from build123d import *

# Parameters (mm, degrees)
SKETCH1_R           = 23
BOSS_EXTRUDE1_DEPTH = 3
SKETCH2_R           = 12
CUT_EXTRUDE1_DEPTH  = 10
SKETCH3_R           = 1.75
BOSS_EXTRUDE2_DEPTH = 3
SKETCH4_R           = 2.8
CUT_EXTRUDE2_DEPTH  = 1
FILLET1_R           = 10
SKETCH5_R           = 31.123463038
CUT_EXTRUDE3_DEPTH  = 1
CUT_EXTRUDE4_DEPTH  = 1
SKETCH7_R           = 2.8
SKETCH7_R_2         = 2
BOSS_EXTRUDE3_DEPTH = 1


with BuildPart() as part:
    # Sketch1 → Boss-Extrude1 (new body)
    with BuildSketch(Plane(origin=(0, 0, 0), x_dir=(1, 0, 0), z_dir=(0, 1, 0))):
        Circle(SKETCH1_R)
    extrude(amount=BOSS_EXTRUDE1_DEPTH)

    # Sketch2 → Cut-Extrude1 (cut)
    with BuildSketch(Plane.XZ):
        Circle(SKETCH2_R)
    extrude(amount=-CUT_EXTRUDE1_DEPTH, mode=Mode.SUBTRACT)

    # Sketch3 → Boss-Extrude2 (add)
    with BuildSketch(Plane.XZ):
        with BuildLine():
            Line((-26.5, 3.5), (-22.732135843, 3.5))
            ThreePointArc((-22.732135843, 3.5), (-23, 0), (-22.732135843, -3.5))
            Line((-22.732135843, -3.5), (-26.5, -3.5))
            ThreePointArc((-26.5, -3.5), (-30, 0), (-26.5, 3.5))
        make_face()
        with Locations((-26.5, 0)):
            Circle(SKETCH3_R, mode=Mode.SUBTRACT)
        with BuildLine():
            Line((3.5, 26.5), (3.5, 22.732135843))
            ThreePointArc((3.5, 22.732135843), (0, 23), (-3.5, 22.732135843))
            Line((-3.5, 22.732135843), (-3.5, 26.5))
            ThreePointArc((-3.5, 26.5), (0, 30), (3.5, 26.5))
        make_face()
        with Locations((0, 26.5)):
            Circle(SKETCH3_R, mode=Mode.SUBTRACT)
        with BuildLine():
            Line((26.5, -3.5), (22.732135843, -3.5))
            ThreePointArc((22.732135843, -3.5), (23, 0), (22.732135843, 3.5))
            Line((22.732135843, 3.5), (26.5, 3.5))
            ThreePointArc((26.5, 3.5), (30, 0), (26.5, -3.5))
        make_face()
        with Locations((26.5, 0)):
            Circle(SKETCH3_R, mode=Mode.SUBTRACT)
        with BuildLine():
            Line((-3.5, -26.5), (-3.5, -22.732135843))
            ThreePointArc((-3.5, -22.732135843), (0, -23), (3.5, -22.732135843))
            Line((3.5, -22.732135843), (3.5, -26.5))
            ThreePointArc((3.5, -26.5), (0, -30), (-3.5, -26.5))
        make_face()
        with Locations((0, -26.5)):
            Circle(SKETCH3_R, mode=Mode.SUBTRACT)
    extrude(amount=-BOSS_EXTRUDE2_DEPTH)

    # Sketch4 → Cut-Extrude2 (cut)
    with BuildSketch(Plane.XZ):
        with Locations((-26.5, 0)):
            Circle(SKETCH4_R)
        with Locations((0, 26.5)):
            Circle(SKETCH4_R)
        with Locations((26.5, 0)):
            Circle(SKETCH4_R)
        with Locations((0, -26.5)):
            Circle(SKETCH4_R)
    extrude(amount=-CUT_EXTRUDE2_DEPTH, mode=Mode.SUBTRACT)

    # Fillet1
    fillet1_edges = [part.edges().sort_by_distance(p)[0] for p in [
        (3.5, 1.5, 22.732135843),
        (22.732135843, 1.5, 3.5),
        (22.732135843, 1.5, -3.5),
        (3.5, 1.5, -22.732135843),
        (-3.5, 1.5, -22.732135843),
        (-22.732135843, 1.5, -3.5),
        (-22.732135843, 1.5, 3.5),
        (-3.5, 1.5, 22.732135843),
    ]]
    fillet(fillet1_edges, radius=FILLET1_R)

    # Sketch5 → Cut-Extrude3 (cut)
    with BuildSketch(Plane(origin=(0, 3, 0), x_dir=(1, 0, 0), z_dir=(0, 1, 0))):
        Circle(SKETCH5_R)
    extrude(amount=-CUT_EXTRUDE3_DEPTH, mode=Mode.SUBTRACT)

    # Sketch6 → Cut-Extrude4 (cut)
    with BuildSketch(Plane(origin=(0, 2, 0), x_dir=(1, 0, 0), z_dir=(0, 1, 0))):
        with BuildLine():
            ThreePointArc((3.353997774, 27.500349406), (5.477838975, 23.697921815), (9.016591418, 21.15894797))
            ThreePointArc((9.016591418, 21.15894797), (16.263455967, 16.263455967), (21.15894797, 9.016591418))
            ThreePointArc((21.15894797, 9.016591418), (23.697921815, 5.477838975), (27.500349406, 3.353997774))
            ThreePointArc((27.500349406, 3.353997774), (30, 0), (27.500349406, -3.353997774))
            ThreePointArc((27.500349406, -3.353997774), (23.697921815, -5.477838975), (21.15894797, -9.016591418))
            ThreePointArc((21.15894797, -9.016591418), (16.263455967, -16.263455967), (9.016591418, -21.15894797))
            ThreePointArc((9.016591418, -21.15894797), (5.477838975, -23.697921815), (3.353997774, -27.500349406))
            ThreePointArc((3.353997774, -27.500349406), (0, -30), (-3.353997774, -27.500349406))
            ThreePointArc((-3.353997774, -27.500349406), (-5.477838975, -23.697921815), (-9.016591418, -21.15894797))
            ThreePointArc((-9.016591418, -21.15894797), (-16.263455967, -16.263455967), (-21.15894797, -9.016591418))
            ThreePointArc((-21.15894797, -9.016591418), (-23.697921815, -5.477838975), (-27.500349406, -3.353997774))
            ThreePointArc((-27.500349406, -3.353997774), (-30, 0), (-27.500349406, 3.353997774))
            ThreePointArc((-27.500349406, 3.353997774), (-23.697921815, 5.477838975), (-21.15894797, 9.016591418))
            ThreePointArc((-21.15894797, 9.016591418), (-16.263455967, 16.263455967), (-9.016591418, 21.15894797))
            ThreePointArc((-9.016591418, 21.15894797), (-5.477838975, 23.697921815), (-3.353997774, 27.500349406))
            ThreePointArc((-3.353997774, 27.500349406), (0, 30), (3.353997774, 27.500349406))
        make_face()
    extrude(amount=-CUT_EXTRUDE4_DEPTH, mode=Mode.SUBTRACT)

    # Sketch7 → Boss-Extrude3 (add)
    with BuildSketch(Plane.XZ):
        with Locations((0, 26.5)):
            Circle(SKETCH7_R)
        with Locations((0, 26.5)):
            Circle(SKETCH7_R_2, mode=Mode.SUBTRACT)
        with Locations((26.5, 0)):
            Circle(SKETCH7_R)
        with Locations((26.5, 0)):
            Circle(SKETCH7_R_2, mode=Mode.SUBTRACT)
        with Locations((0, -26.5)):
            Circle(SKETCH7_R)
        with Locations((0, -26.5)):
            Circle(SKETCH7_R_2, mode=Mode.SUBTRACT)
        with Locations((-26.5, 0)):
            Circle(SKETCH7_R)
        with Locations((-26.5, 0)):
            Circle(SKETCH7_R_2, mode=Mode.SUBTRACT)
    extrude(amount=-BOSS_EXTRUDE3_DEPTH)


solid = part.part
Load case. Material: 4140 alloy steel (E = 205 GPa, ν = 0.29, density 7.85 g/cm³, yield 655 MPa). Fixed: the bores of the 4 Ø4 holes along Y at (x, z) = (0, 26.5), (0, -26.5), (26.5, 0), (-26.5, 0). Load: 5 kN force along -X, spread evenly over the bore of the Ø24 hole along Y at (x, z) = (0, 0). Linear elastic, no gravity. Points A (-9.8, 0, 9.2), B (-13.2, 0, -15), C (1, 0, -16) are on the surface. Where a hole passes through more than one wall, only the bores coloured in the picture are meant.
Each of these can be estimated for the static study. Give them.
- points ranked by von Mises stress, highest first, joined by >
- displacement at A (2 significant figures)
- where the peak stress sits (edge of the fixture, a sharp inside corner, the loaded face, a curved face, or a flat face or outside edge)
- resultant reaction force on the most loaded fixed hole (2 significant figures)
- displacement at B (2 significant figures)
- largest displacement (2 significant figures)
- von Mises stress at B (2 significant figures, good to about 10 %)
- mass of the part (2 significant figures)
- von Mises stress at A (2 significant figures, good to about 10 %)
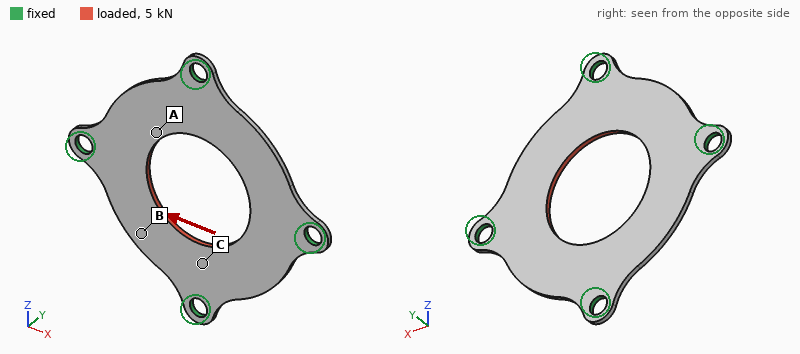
A > B > C
15 µm
edge of the fixture
1.7 kN
14 µm
18 µm
62 MPa
11 g
110 MPa
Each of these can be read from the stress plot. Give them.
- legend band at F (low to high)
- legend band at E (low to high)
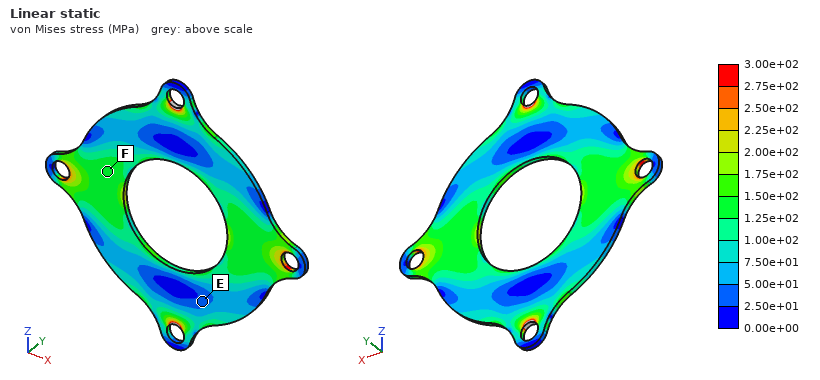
1.25e+02 to 1.50e+02 MPa
2.50e+01 to 5.00e+01 MPa
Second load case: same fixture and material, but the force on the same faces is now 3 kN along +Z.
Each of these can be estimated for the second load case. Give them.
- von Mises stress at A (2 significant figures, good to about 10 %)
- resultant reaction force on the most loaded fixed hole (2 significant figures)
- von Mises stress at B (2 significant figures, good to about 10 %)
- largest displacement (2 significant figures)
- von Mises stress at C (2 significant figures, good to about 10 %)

64 MPa
1.0 kN
34 MPa
11 µm
78 MPa
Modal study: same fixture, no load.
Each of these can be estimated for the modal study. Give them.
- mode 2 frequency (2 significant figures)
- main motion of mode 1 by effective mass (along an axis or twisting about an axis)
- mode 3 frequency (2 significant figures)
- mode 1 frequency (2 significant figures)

4400 Hz
along Y
4400 Hz
3600 Hz
